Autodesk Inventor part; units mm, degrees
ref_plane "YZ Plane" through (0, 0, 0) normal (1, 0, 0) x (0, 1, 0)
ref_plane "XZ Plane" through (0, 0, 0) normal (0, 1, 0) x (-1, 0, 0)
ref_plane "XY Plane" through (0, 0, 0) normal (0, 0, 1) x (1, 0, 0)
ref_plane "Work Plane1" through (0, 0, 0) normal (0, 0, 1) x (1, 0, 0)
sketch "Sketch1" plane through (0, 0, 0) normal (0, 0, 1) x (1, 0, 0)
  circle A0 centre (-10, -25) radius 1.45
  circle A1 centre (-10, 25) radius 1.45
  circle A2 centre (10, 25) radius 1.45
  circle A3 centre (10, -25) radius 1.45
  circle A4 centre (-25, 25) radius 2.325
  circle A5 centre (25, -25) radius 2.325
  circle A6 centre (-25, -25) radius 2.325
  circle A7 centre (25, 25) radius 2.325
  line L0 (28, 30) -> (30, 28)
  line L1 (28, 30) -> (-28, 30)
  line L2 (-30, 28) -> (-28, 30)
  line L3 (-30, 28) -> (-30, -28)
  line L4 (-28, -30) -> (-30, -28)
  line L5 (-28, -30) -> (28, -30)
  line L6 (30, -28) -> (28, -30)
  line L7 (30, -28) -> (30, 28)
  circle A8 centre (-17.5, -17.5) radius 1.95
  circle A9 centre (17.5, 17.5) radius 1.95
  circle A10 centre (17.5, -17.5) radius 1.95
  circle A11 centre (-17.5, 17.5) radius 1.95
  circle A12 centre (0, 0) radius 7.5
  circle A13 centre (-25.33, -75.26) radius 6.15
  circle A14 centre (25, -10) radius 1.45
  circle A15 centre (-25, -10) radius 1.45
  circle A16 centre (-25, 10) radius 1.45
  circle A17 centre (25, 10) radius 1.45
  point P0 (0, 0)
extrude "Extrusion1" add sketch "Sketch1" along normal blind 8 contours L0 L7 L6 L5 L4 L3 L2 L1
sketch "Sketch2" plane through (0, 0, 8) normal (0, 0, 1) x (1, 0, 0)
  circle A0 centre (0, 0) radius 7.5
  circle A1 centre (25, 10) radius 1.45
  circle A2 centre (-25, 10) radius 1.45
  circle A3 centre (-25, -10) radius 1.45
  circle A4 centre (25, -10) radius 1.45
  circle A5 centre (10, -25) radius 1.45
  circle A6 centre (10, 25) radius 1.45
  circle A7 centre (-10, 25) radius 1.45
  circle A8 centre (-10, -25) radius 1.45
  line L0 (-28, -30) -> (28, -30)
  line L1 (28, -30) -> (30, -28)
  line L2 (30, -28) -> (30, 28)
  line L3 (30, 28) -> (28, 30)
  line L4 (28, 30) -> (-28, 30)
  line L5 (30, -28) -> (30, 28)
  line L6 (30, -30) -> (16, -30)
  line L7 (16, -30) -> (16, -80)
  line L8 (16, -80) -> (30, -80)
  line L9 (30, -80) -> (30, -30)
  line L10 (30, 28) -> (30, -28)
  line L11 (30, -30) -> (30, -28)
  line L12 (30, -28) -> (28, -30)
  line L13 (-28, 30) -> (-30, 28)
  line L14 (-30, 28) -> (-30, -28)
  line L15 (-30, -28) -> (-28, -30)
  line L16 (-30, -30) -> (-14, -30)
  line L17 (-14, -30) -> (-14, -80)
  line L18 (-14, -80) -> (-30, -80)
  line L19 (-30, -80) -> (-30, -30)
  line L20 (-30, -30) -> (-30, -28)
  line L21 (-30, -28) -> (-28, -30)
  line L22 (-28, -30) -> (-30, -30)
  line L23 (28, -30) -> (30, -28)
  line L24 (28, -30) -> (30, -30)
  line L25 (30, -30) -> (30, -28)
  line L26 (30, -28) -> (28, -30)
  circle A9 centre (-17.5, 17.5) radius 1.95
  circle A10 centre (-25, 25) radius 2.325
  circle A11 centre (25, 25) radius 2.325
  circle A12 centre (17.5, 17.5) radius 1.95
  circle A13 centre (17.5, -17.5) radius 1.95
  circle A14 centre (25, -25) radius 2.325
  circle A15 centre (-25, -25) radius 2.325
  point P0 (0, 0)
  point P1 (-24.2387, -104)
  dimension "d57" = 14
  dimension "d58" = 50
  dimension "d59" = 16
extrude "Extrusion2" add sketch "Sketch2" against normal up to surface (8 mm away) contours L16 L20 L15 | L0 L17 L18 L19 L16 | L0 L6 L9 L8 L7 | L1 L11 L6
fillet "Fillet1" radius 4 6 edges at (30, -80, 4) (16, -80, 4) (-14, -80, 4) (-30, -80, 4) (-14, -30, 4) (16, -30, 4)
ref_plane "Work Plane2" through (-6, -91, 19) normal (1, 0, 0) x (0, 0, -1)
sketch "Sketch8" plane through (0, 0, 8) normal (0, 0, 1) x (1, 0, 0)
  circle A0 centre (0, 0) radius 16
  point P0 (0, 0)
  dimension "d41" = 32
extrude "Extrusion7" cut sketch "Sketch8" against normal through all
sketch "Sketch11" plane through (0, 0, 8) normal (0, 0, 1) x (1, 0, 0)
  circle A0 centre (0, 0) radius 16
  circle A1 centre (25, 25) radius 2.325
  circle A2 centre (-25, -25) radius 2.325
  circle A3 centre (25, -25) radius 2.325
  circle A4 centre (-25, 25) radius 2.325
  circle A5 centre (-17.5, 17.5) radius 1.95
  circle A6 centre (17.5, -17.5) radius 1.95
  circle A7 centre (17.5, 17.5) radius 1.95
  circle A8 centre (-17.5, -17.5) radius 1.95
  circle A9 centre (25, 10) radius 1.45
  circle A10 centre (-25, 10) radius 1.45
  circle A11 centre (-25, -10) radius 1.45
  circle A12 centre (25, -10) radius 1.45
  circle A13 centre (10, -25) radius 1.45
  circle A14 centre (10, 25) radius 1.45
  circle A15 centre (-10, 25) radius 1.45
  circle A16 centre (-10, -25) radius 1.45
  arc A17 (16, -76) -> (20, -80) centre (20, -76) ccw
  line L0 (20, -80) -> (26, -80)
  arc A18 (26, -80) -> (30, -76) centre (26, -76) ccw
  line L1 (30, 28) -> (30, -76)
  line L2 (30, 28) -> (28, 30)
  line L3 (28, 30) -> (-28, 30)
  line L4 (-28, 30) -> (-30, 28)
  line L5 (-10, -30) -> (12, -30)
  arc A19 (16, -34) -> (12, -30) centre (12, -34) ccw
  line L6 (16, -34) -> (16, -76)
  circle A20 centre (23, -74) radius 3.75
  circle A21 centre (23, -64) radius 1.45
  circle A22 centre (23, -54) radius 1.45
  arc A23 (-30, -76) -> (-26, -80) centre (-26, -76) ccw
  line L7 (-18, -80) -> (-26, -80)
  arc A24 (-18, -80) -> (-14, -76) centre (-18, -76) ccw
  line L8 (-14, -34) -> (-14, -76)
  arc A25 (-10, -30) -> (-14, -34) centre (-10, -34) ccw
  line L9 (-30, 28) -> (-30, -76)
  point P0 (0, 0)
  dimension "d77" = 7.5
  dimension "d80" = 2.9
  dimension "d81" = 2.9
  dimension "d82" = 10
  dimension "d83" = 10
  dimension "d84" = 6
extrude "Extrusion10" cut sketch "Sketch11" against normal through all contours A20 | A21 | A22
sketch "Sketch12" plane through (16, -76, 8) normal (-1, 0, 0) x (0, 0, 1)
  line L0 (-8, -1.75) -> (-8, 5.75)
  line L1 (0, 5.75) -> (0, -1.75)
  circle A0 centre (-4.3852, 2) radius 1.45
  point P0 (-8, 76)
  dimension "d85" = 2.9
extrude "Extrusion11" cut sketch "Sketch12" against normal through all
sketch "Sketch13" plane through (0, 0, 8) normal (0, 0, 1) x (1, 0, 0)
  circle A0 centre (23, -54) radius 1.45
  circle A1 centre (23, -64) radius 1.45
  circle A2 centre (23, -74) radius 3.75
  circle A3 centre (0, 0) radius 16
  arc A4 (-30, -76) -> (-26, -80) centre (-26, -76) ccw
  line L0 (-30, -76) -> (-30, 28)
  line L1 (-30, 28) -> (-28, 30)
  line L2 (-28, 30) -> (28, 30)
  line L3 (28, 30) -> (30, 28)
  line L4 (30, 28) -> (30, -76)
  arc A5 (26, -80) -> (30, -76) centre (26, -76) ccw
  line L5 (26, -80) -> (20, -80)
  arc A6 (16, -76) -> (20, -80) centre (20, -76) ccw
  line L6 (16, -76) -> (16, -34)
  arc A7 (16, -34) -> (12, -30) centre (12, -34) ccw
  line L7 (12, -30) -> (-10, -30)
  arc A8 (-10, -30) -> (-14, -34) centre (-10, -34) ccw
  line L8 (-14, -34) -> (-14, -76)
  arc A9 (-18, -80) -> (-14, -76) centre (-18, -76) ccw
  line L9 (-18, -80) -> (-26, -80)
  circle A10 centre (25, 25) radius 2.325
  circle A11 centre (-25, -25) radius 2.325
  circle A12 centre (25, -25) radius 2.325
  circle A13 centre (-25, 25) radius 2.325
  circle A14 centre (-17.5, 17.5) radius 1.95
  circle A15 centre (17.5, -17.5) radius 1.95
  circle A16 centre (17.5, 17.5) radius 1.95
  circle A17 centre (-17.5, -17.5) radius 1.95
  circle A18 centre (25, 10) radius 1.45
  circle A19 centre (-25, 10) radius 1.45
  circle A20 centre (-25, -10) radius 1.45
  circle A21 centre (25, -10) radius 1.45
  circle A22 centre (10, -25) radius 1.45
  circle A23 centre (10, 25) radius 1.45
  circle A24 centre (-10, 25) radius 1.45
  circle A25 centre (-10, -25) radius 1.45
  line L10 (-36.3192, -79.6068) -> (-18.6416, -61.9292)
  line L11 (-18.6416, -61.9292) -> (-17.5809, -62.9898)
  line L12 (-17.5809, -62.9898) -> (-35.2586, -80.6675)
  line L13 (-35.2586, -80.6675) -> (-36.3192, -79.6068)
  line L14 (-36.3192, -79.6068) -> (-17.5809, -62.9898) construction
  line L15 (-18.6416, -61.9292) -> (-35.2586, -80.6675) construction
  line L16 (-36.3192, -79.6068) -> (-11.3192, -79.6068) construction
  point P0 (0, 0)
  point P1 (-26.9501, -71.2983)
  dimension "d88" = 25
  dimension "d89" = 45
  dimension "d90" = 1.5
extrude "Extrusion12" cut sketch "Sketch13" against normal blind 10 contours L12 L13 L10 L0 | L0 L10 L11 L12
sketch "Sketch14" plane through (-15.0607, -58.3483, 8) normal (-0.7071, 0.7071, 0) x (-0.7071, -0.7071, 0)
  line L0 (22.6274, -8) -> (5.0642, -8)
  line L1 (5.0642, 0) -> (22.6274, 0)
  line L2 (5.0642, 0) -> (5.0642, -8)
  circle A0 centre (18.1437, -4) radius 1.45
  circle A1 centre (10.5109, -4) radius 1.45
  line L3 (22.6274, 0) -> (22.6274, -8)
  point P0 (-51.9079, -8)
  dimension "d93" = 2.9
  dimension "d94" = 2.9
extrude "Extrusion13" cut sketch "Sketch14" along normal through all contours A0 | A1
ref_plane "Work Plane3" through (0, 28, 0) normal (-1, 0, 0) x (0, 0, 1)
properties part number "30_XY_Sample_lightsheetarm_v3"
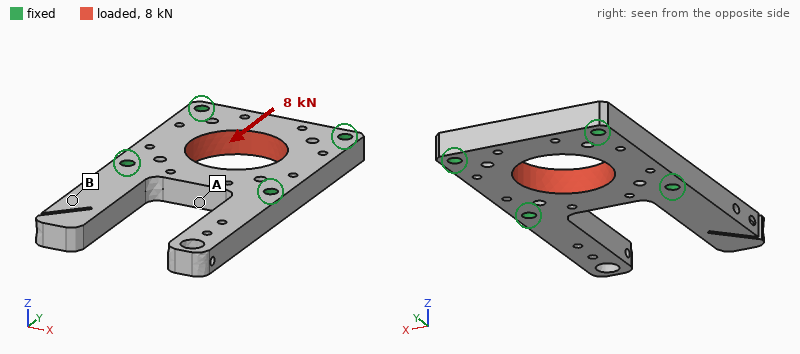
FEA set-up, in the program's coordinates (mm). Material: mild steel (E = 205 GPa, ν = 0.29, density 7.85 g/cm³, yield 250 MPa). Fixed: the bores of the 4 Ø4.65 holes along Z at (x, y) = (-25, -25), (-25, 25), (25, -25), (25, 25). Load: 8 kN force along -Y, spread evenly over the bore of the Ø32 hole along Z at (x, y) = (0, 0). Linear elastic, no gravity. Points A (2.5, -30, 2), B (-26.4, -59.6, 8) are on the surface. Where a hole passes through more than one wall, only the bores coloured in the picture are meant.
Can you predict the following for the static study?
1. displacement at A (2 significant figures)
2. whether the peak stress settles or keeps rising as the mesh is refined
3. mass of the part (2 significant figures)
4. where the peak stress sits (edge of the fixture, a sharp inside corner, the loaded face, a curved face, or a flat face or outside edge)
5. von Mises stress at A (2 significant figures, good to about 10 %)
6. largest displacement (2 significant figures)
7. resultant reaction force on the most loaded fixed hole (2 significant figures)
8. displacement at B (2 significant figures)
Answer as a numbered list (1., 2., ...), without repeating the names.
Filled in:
1. 3.4 µm
2. keeps rising
3. 250 g
4. edge of the fixture
5. 17 MPa
6. 8.1 µm
7. 2.2 kN
8. 5.0 µm
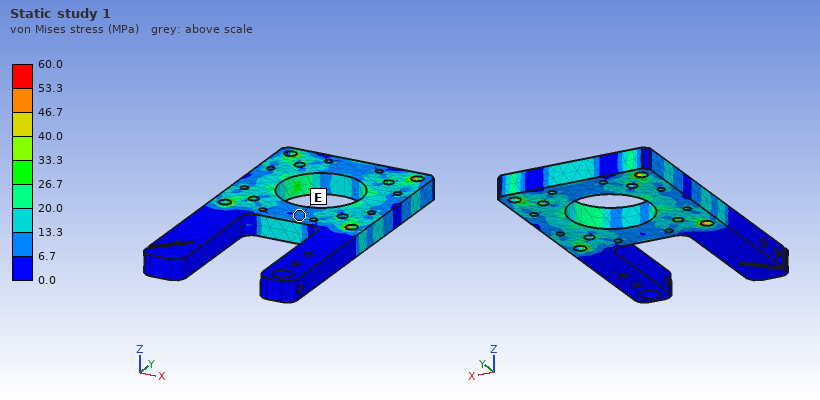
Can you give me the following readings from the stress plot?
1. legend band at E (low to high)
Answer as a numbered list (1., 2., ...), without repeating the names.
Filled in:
1. 6.7 to 13.3 MPa
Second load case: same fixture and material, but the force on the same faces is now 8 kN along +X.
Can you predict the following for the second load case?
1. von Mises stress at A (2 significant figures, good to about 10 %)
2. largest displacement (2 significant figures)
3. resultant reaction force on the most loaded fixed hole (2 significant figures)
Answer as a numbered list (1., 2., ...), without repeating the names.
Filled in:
1. 5.4 MPa
2. 4.1 µm
3. 2.2 kN
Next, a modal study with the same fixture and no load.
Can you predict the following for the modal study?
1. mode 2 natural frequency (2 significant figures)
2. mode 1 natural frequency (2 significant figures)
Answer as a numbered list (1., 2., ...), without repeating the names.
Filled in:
1. 2500 Hz
2. 2200 Hz
